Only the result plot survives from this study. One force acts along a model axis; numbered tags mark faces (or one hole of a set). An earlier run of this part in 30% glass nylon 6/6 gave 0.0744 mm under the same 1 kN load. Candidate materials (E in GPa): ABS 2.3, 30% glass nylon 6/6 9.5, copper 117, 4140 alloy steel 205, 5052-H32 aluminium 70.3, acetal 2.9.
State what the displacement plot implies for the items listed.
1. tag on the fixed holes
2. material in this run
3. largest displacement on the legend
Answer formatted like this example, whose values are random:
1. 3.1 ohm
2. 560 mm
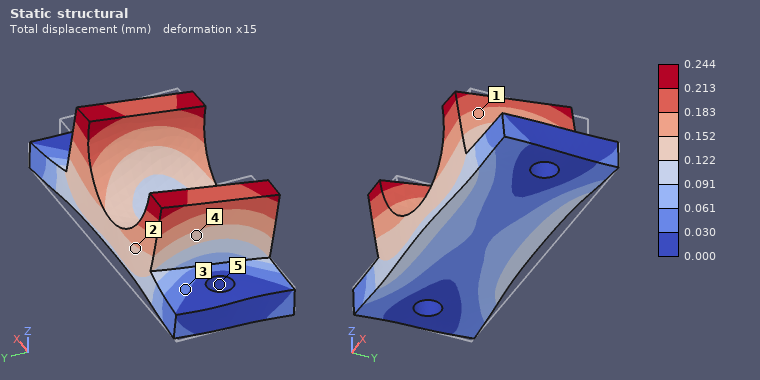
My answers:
1. 5
2. acetal
3. 0.244 mm
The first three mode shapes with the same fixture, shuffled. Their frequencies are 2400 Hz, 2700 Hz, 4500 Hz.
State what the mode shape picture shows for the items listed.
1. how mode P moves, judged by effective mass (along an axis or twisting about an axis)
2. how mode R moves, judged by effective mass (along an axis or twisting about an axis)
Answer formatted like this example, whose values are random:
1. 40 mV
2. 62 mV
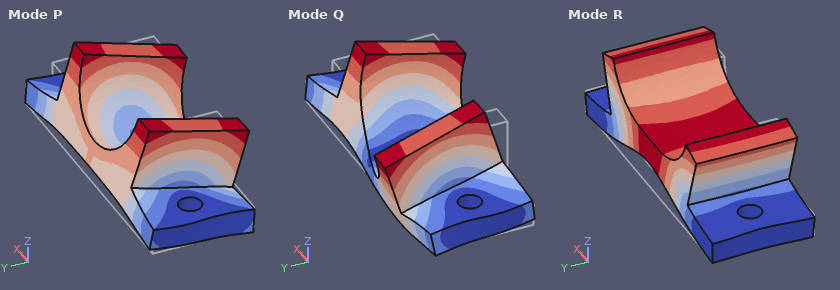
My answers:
1. along Y
2. along Z
